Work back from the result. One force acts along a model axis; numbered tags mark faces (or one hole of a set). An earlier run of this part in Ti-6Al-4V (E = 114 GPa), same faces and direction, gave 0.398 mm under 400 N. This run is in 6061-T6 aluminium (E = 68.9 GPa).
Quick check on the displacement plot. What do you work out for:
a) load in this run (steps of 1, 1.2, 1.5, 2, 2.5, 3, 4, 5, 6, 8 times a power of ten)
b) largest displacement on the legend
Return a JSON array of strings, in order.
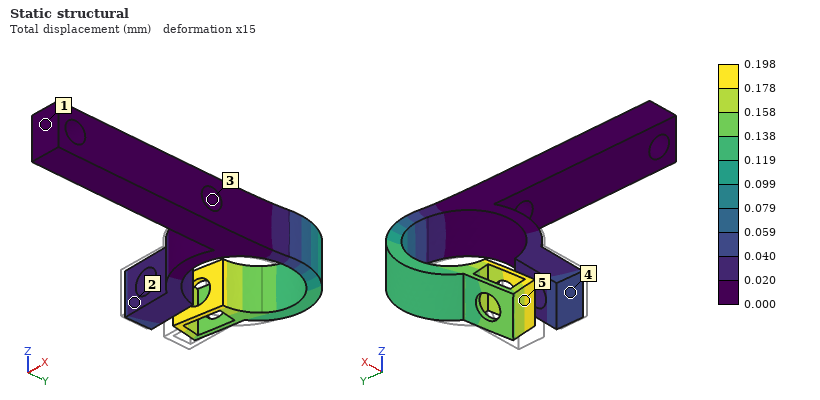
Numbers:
["120 N", "0.198 mm"]
